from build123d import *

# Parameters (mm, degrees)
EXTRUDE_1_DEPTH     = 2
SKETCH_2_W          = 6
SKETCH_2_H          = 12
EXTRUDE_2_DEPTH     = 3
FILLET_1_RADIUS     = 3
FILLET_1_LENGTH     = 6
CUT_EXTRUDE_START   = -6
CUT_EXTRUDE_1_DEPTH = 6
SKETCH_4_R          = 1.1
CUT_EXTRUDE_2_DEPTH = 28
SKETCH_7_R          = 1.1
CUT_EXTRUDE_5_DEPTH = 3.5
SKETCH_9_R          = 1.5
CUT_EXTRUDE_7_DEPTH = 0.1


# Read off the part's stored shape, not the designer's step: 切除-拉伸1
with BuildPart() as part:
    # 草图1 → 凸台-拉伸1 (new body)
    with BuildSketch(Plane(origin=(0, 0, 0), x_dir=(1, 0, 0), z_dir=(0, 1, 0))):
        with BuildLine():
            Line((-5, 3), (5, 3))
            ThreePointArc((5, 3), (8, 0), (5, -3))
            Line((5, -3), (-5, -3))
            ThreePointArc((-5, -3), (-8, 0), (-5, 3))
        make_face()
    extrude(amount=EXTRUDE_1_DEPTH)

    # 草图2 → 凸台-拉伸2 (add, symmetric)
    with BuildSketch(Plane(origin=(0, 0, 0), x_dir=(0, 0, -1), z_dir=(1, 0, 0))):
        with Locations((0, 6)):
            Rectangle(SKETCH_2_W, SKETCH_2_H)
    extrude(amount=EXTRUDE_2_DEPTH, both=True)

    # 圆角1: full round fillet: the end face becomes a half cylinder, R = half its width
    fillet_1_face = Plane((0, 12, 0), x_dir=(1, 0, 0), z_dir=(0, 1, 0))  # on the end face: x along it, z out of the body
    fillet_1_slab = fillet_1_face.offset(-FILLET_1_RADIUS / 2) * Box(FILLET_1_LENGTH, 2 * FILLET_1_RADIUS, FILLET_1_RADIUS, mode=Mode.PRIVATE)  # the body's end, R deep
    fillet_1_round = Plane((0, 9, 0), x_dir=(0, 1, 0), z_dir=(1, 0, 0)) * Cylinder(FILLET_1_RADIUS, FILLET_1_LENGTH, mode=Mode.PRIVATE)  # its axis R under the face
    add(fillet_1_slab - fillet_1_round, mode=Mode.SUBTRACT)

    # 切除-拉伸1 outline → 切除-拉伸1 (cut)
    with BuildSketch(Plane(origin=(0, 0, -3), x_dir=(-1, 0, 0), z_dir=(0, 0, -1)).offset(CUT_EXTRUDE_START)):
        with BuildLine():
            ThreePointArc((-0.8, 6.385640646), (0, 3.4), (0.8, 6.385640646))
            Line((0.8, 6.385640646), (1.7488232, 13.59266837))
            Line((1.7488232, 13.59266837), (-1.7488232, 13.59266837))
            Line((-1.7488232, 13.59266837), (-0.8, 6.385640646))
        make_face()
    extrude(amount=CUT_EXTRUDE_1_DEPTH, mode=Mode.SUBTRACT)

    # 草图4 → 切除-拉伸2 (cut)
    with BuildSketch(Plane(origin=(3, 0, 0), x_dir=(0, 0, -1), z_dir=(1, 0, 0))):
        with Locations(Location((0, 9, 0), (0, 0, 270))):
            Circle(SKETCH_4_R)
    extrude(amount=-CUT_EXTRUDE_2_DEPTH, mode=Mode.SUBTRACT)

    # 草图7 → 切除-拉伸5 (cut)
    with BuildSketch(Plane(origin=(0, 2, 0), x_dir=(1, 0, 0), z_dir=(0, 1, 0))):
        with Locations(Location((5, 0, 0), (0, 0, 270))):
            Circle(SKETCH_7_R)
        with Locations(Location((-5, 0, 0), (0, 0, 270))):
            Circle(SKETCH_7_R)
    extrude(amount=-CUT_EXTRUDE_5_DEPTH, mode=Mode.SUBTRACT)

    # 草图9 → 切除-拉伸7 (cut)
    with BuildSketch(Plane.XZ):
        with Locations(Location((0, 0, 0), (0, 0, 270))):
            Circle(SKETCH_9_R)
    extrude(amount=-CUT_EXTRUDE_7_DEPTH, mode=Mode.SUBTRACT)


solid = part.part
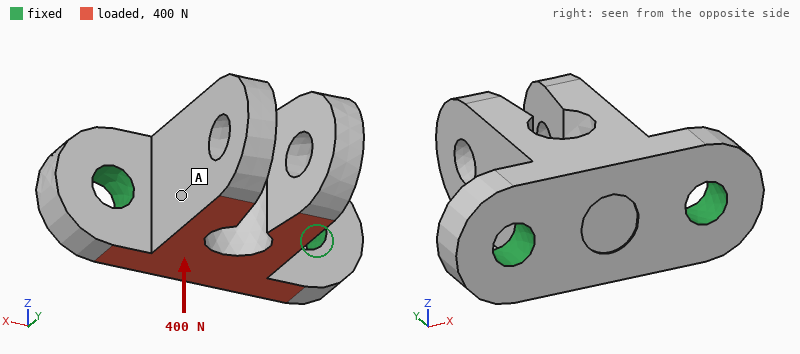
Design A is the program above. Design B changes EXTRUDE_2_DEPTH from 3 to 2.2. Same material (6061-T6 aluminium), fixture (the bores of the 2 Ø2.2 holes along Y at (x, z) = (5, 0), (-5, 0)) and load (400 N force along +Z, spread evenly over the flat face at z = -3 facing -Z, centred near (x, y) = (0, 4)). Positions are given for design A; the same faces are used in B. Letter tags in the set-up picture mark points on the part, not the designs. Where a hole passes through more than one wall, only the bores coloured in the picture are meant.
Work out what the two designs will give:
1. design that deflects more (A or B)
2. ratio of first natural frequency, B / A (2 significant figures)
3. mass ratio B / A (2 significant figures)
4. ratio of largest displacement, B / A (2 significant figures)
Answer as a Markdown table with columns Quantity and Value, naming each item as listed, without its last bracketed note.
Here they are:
| Quantity | Value |
|---|---|
| design that deflects more | B |
| ratio of first natural frequency, B / A | 0.53 |
| mass ratio B / A | 0.77 |
| ratio of largest displacement, B / A | 1.1 |
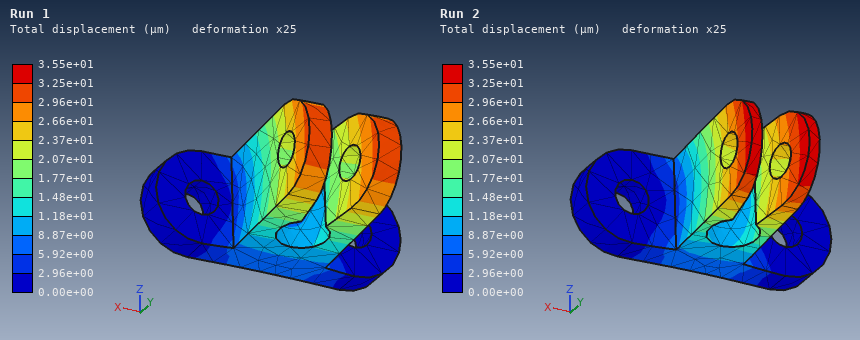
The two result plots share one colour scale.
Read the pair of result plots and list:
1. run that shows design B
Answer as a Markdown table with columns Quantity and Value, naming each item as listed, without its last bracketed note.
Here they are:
| Quantity | Value |
|---|---|
| run that shows design B | Run 2 |
